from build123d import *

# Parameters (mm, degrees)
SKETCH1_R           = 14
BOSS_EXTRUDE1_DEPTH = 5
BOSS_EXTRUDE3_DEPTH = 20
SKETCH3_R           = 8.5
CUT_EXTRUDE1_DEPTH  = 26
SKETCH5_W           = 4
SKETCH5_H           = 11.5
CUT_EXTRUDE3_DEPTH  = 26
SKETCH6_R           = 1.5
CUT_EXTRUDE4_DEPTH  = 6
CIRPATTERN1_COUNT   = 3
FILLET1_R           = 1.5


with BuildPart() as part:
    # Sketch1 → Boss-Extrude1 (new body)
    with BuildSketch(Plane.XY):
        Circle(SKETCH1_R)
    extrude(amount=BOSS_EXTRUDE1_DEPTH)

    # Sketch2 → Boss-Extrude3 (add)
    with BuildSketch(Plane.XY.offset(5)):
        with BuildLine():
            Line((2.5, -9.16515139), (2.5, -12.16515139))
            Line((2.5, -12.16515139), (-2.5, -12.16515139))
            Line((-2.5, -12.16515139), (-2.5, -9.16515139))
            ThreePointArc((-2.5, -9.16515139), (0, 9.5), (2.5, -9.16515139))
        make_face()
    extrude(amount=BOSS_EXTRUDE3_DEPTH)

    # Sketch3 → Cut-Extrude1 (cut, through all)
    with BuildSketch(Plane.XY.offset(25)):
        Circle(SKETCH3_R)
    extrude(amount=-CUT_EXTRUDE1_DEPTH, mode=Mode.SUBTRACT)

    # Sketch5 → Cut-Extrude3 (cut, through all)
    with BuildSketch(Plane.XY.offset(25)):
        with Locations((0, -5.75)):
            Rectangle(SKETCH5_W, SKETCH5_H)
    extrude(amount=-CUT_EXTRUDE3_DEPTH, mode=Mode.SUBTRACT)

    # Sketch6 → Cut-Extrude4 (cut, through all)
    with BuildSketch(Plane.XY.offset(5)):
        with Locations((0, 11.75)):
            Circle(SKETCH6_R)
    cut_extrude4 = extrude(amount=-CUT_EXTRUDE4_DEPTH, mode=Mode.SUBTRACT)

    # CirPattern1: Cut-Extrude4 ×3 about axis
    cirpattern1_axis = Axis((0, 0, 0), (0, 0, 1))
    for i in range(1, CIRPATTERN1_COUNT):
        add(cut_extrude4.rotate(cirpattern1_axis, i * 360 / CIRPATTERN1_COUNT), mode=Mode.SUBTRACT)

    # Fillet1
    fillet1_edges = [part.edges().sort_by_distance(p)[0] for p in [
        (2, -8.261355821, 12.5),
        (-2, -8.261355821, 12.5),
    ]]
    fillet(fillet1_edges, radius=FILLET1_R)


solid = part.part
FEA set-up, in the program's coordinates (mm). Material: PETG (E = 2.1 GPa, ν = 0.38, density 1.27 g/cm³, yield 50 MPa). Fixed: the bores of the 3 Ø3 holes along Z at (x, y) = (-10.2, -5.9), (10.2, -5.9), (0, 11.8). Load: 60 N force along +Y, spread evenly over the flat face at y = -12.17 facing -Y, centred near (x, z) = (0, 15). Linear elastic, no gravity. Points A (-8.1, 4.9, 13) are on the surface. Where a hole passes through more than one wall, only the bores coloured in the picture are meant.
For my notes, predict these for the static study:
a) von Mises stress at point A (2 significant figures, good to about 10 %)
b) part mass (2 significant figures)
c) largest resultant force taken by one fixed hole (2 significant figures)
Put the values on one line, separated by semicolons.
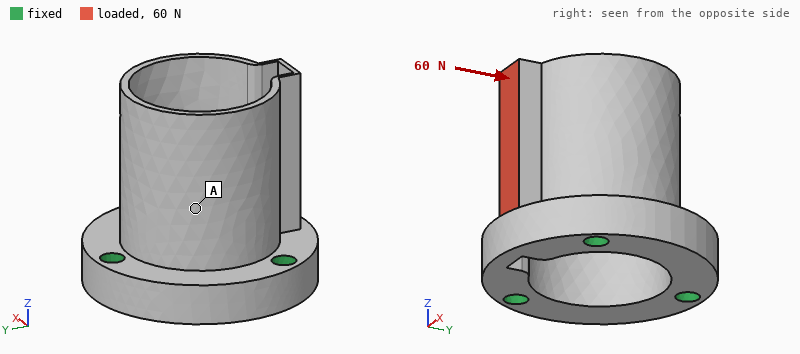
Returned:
2.2 MPa; 3.7 g; 36 N
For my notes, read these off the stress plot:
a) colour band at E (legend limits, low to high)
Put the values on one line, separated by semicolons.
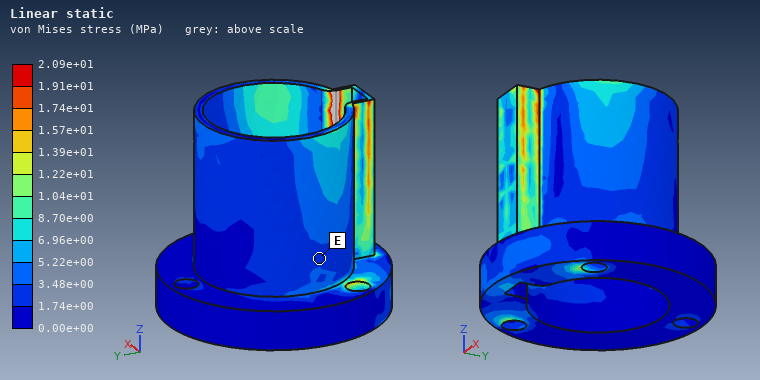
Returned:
1.74e+00 to 3.48e+00 MPa
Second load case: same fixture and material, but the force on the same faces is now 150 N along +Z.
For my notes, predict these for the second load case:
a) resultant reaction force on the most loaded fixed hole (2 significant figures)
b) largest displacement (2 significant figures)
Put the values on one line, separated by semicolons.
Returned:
84 N; 0.51 mm
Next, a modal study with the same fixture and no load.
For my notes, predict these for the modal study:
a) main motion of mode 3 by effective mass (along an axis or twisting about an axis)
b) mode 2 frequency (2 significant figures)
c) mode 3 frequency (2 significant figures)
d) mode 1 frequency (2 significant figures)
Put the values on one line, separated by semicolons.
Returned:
along Y; 3100 Hz; 3700 Hz; 2400 Hz
